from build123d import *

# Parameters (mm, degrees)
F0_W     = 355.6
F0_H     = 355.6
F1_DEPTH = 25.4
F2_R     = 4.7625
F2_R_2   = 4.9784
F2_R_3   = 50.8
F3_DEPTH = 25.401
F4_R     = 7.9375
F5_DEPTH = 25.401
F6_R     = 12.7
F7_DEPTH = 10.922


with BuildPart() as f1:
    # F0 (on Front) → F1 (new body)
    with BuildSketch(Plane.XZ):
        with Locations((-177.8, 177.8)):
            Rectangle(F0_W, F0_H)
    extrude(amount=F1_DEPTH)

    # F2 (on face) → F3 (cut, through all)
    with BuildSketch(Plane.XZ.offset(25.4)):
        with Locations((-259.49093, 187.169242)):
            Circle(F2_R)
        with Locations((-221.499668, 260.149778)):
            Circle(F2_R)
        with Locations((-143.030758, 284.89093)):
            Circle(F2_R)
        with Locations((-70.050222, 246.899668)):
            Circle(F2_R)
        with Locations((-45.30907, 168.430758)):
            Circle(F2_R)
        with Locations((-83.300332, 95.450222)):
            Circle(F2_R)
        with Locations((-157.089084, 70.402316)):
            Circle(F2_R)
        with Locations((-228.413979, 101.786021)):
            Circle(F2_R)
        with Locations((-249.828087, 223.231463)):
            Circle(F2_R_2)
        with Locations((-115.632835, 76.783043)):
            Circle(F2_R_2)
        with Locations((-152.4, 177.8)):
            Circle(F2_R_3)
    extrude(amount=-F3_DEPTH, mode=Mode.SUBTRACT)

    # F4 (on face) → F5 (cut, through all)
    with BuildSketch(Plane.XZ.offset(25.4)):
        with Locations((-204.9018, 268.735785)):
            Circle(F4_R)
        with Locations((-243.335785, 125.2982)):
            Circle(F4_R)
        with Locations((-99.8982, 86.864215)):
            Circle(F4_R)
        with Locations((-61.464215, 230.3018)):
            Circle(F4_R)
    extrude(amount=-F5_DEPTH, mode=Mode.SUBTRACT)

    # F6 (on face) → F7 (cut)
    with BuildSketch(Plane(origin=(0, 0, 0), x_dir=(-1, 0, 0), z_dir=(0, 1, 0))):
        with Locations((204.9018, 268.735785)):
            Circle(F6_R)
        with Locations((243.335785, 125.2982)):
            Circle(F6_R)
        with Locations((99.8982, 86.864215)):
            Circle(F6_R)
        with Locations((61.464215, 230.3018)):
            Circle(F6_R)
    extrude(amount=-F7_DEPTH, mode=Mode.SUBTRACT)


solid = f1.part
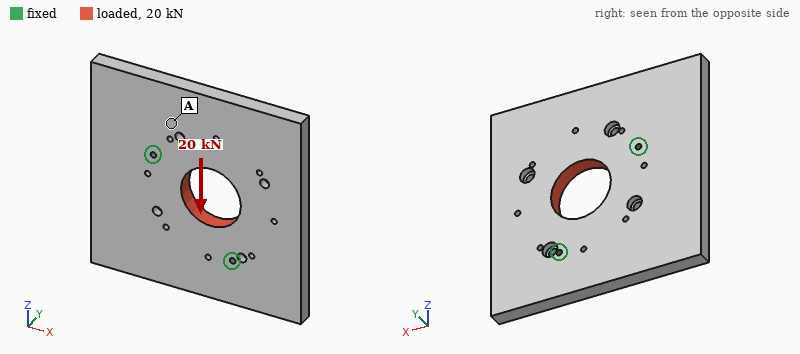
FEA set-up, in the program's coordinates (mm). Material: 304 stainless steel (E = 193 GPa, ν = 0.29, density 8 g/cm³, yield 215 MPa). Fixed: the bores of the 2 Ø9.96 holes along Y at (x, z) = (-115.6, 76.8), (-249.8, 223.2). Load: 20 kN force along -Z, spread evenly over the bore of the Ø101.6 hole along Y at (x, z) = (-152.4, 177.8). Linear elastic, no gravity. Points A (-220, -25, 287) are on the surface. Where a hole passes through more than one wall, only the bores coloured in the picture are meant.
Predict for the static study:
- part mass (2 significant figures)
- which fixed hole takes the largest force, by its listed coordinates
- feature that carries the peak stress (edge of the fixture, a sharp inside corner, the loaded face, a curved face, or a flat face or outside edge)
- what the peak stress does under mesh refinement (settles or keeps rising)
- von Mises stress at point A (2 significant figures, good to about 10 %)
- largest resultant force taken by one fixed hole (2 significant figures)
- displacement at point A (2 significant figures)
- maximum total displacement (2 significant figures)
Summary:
24 kg
(-115.6, 76.8)
edge of the fixture
keeps rising
2.1 MPa
12 kN
2.8 µm
5.9 µm
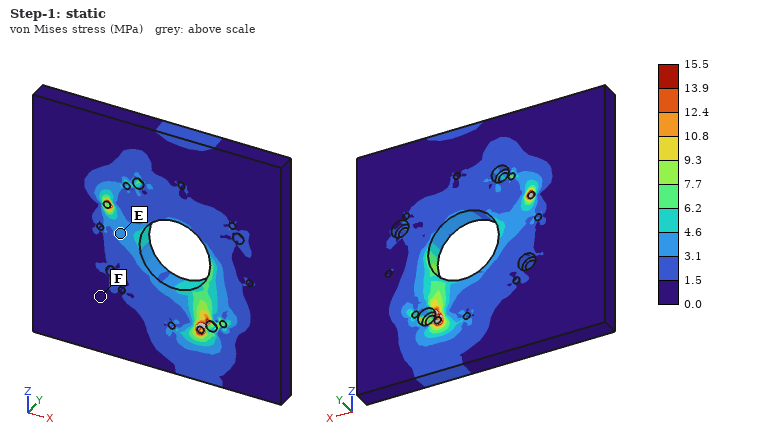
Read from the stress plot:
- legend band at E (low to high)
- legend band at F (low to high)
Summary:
3.1 to 4.6 MPa
0.0 to 1.5 MPa
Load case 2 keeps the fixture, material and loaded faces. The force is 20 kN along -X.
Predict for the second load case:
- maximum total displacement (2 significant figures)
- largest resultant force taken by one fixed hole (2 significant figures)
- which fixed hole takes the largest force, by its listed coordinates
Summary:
5.2 µm
13 kN
(-249.8, 223.2)
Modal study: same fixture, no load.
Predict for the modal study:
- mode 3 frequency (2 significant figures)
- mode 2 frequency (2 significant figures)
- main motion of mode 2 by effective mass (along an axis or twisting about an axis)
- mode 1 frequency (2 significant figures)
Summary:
820 Hz
550 Hz
along Y
310 Hz
